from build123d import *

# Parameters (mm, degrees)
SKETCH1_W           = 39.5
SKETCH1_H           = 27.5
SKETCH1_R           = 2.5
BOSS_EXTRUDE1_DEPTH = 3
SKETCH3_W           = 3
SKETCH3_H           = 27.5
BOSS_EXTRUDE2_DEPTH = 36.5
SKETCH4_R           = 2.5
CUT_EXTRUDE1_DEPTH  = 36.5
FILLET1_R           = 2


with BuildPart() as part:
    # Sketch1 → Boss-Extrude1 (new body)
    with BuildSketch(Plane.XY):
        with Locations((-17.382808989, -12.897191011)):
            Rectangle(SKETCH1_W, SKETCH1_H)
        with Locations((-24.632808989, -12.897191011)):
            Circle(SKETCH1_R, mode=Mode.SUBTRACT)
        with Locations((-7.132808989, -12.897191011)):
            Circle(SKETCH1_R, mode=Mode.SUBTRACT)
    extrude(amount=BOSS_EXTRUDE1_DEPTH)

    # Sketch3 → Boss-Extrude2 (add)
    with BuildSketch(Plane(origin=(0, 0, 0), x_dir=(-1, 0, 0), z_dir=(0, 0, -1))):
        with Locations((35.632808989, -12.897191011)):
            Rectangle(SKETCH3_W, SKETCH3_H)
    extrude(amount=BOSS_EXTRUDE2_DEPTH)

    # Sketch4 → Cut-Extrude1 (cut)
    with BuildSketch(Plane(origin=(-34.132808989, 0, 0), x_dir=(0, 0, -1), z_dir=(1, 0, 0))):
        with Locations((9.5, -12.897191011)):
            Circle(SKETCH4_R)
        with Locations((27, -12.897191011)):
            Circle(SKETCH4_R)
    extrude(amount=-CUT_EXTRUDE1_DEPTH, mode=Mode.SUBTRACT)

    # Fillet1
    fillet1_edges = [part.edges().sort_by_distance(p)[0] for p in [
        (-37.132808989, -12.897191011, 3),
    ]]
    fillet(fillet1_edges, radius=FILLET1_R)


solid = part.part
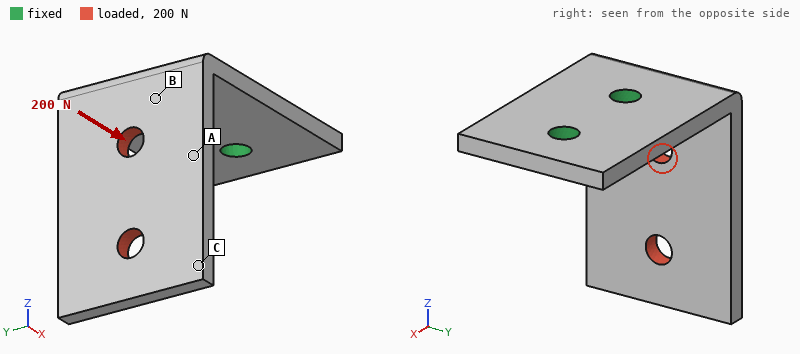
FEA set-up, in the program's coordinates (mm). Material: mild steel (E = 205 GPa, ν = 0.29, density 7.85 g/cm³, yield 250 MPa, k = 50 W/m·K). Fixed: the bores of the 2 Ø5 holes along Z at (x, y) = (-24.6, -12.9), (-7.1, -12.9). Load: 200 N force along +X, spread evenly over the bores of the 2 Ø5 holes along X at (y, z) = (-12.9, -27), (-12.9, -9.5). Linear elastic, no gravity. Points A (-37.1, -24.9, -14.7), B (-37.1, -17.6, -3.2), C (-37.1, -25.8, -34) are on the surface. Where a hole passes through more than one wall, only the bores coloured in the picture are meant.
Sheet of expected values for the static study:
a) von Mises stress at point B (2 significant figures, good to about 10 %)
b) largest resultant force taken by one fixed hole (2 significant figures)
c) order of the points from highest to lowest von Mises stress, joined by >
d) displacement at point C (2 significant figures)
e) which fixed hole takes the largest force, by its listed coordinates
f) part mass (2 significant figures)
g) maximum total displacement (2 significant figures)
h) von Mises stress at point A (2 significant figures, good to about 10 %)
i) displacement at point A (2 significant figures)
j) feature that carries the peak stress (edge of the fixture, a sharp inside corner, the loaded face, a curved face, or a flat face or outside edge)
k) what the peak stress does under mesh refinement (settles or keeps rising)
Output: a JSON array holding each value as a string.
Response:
["67 MPa", "180 N", "B > A > C", "0.21 mm", "(-24.6, -12.9)", "47 g", "0.23 mm", "34 MPa", "0.081 mm", "edge of the fixture", "keeps rising"]
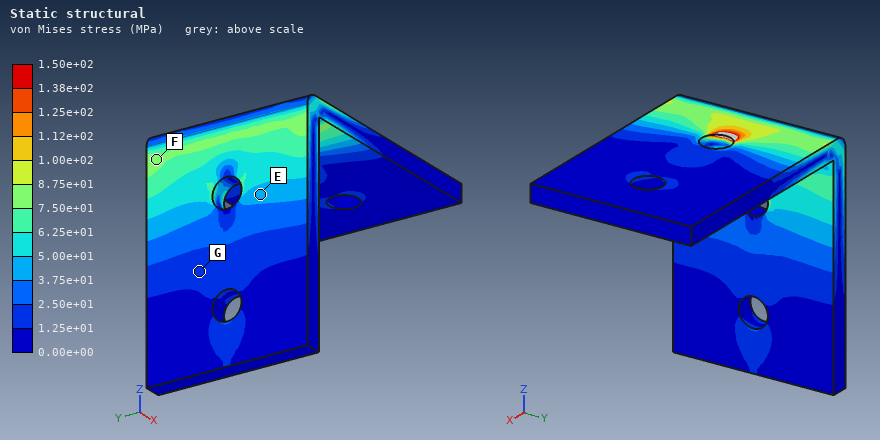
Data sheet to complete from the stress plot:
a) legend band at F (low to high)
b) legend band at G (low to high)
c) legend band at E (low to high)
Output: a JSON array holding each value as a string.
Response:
["7.50e+01 to 8.75e+01 MPa", "1.25e+01 to 2.50e+01 MPa", "3.75e+01 to 5.00e+01 MPa"]
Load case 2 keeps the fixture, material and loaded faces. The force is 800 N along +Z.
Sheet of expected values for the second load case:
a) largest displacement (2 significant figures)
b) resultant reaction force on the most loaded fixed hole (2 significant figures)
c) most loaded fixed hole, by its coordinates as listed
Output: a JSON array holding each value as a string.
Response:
["0.14 mm", "910 N", "(-24.6, -12.9)"]
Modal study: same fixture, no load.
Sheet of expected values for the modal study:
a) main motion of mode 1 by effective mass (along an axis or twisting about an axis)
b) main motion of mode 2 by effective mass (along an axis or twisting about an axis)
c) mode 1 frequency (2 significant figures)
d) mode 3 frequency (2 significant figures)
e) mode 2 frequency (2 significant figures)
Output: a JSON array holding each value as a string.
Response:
["along X", "along Y", "1200 Hz", "4800 Hz", "2100 Hz"]
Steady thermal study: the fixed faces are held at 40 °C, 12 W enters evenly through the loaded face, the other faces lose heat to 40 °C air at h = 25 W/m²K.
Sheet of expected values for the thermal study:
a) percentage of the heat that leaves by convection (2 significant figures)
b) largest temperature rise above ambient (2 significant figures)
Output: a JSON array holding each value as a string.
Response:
["29 %", "75 K"]
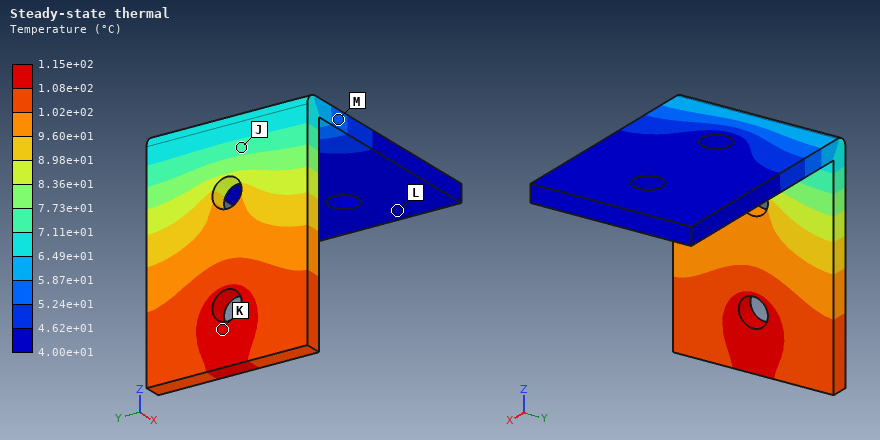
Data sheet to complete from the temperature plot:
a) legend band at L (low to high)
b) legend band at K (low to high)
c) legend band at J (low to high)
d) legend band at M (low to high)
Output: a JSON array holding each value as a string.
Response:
["4.00e+01 to 4.62e+01 °C", "1.08e+02 to 1.15e+02 °C", "7.11e+01 to 7.73e+01 °C", "5.24e+01 to 5.87e+01 °C"]
